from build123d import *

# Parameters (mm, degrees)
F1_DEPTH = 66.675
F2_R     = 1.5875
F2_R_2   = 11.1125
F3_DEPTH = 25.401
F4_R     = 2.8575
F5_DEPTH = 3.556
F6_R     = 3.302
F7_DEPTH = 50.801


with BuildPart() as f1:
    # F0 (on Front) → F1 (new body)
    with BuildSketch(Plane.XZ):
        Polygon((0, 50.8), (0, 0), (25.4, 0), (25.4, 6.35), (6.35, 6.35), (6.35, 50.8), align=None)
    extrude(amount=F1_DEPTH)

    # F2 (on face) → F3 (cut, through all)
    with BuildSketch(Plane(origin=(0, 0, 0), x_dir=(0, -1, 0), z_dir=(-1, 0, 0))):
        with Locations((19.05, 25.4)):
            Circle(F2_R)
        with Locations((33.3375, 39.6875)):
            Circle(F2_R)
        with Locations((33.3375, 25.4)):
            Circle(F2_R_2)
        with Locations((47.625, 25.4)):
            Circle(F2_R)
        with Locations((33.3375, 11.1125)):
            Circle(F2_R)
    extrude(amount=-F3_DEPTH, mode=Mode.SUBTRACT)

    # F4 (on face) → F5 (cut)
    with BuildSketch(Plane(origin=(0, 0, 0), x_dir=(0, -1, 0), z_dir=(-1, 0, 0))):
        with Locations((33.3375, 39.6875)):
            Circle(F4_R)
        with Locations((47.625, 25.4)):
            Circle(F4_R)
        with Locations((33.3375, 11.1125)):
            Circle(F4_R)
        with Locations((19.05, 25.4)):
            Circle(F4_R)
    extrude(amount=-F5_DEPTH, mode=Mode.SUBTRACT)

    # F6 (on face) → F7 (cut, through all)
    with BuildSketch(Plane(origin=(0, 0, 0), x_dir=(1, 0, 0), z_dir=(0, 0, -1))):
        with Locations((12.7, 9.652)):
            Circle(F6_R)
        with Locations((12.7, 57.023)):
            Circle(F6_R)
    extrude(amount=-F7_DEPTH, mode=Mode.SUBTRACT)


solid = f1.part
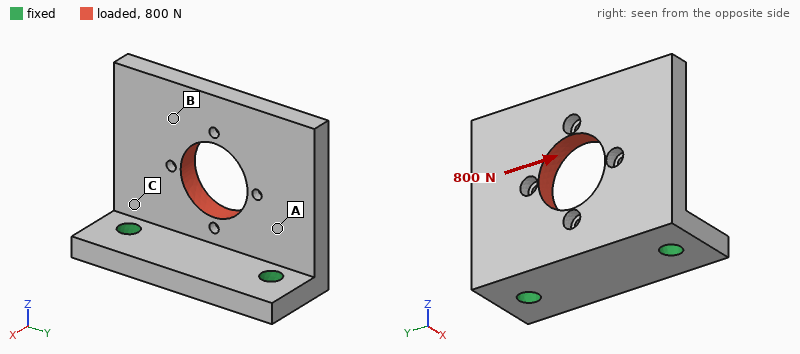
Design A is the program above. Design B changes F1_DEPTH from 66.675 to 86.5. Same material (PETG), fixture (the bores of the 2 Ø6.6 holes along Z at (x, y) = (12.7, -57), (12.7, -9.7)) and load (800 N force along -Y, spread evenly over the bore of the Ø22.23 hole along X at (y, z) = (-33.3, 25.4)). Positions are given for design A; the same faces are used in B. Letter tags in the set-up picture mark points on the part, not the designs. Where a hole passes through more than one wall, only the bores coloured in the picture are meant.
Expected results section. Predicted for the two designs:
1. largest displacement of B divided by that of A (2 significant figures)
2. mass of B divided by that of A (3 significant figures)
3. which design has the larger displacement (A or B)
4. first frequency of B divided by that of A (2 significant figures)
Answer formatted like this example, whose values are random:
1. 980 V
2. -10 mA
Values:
1. 1.2
2. 1.34
3. B
4. 0.97
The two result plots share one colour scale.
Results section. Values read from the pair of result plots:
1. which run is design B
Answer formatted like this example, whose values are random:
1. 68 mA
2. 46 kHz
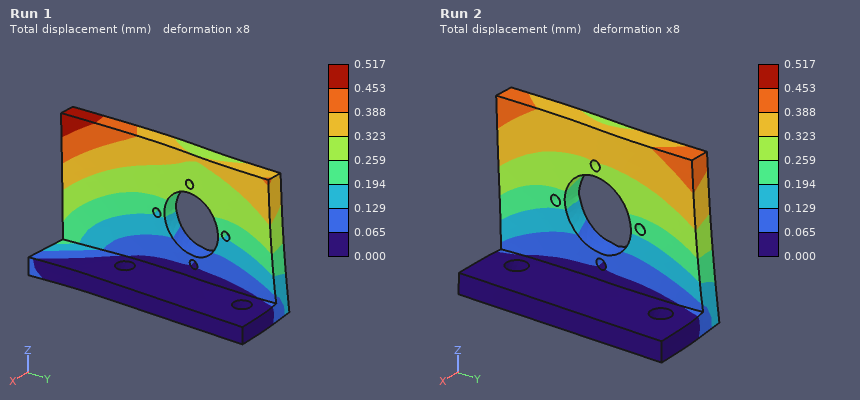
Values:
1. Run 1
